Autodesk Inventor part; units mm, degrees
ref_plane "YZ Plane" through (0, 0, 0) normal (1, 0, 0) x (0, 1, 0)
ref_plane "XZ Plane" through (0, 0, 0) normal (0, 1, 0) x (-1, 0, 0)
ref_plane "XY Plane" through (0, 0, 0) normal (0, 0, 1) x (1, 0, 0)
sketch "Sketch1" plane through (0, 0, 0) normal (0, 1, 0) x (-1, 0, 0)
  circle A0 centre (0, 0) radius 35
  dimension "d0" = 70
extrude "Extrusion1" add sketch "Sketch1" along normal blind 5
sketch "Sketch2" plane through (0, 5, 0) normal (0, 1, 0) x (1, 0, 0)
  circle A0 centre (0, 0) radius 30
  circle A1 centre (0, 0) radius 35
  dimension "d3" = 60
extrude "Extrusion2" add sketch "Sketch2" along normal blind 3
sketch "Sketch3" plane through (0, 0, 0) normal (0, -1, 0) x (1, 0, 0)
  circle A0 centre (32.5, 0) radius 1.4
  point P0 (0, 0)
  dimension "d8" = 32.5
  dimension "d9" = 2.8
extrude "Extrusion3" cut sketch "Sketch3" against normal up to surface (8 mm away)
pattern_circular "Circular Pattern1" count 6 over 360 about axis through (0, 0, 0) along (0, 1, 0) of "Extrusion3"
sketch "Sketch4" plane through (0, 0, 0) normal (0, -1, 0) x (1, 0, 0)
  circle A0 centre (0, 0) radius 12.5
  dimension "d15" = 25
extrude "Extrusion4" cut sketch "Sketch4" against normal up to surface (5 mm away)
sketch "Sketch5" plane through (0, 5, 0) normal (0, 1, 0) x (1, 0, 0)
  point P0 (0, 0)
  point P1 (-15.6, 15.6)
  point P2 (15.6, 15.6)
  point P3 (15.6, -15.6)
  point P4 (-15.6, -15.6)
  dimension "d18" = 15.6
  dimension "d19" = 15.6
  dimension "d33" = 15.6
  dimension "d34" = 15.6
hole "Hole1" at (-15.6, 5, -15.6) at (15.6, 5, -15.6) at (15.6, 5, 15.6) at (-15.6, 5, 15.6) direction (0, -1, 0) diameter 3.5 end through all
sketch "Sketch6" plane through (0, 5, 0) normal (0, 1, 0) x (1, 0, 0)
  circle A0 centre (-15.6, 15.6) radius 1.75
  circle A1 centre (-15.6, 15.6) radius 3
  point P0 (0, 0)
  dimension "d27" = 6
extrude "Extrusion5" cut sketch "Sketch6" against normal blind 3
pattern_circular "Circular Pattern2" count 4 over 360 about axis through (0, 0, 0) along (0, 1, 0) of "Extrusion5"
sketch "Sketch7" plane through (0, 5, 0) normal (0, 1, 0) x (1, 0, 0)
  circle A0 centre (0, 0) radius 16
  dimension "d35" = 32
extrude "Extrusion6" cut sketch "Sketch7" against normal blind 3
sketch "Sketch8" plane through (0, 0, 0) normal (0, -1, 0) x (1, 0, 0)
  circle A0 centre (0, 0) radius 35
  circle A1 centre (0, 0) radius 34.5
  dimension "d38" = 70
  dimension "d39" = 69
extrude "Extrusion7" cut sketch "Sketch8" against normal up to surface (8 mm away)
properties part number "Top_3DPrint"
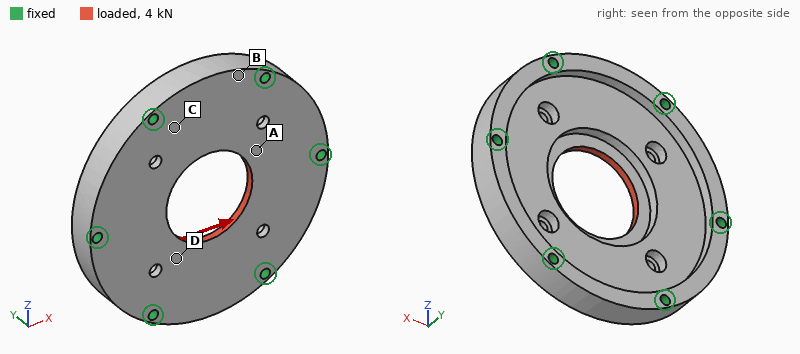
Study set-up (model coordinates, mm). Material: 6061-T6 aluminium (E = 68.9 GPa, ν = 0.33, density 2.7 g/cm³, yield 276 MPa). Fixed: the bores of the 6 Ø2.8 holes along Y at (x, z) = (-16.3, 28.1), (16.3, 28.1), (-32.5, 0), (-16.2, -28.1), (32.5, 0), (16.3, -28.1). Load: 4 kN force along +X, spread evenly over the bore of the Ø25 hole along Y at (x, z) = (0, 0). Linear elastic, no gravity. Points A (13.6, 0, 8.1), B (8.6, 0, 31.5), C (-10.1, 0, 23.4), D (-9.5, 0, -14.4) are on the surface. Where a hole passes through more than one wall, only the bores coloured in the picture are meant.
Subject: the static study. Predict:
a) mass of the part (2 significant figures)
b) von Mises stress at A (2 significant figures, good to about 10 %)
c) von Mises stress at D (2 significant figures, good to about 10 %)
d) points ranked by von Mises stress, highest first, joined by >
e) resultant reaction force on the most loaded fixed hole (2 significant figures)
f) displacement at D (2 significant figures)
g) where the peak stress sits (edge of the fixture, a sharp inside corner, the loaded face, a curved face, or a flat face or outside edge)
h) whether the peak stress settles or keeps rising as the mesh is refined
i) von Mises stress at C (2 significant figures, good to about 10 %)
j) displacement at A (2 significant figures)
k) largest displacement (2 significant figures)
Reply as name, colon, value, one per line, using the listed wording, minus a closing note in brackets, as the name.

mass of the part: 47 g
von Mises stress at A: 24 MPa
von Mises stress at D: 18 MPa
points ranked by von Mises stress, highest first, joined by >: A > D > C > B
resultant reaction force on the most loaded fixed hole: 930 N
displacement at D: 4.7 µm
where the peak stress sits: edge of the fixture
whether the peak stress settles or keeps rising as the mesh is refined: keeps rising
von Mises stress at C: 9.4 MPa
displacement at A: 7.8 µm
largest displacement: 12 µm
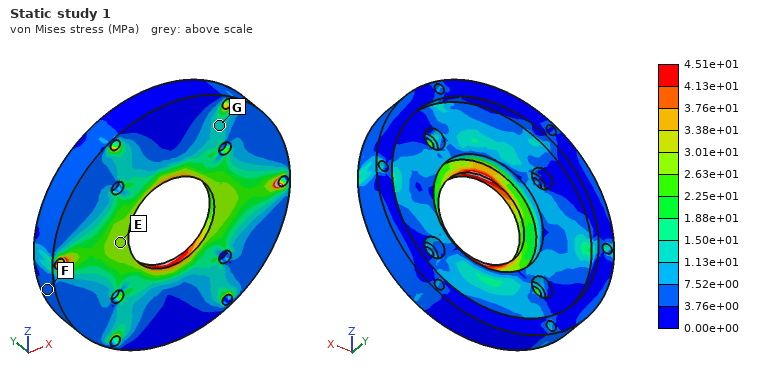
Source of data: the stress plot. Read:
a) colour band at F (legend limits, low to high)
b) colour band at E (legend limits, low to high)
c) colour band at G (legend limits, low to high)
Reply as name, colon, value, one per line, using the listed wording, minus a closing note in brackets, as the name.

colour band at F: 3.76e+00 to 7.52e+00 MPa
colour band at E: 2.63e+01 to 3.01e+01 MPa
colour band at G: 1.13e+01 to 1.50e+01 MPa
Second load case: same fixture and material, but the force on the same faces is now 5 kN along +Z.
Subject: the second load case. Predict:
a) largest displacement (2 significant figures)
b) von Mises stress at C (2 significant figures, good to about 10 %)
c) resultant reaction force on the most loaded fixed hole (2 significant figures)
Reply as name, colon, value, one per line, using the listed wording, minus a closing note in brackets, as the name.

largest displacement: 15 µm
von Mises stress at C: 25 MPa
resultant reaction force on the most loaded fixed hole: 1.0 kN
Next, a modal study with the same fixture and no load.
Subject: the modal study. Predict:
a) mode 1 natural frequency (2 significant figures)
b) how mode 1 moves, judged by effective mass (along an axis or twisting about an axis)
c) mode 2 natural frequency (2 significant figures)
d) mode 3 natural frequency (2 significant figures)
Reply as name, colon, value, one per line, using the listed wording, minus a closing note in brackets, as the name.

mode 1 natural frequency: 13 kHz
how mode 1 moves, judged by effective mass: along Y
mode 2 natural frequency: 16 kHz
mode 3 natural frequency: 16 kHz
